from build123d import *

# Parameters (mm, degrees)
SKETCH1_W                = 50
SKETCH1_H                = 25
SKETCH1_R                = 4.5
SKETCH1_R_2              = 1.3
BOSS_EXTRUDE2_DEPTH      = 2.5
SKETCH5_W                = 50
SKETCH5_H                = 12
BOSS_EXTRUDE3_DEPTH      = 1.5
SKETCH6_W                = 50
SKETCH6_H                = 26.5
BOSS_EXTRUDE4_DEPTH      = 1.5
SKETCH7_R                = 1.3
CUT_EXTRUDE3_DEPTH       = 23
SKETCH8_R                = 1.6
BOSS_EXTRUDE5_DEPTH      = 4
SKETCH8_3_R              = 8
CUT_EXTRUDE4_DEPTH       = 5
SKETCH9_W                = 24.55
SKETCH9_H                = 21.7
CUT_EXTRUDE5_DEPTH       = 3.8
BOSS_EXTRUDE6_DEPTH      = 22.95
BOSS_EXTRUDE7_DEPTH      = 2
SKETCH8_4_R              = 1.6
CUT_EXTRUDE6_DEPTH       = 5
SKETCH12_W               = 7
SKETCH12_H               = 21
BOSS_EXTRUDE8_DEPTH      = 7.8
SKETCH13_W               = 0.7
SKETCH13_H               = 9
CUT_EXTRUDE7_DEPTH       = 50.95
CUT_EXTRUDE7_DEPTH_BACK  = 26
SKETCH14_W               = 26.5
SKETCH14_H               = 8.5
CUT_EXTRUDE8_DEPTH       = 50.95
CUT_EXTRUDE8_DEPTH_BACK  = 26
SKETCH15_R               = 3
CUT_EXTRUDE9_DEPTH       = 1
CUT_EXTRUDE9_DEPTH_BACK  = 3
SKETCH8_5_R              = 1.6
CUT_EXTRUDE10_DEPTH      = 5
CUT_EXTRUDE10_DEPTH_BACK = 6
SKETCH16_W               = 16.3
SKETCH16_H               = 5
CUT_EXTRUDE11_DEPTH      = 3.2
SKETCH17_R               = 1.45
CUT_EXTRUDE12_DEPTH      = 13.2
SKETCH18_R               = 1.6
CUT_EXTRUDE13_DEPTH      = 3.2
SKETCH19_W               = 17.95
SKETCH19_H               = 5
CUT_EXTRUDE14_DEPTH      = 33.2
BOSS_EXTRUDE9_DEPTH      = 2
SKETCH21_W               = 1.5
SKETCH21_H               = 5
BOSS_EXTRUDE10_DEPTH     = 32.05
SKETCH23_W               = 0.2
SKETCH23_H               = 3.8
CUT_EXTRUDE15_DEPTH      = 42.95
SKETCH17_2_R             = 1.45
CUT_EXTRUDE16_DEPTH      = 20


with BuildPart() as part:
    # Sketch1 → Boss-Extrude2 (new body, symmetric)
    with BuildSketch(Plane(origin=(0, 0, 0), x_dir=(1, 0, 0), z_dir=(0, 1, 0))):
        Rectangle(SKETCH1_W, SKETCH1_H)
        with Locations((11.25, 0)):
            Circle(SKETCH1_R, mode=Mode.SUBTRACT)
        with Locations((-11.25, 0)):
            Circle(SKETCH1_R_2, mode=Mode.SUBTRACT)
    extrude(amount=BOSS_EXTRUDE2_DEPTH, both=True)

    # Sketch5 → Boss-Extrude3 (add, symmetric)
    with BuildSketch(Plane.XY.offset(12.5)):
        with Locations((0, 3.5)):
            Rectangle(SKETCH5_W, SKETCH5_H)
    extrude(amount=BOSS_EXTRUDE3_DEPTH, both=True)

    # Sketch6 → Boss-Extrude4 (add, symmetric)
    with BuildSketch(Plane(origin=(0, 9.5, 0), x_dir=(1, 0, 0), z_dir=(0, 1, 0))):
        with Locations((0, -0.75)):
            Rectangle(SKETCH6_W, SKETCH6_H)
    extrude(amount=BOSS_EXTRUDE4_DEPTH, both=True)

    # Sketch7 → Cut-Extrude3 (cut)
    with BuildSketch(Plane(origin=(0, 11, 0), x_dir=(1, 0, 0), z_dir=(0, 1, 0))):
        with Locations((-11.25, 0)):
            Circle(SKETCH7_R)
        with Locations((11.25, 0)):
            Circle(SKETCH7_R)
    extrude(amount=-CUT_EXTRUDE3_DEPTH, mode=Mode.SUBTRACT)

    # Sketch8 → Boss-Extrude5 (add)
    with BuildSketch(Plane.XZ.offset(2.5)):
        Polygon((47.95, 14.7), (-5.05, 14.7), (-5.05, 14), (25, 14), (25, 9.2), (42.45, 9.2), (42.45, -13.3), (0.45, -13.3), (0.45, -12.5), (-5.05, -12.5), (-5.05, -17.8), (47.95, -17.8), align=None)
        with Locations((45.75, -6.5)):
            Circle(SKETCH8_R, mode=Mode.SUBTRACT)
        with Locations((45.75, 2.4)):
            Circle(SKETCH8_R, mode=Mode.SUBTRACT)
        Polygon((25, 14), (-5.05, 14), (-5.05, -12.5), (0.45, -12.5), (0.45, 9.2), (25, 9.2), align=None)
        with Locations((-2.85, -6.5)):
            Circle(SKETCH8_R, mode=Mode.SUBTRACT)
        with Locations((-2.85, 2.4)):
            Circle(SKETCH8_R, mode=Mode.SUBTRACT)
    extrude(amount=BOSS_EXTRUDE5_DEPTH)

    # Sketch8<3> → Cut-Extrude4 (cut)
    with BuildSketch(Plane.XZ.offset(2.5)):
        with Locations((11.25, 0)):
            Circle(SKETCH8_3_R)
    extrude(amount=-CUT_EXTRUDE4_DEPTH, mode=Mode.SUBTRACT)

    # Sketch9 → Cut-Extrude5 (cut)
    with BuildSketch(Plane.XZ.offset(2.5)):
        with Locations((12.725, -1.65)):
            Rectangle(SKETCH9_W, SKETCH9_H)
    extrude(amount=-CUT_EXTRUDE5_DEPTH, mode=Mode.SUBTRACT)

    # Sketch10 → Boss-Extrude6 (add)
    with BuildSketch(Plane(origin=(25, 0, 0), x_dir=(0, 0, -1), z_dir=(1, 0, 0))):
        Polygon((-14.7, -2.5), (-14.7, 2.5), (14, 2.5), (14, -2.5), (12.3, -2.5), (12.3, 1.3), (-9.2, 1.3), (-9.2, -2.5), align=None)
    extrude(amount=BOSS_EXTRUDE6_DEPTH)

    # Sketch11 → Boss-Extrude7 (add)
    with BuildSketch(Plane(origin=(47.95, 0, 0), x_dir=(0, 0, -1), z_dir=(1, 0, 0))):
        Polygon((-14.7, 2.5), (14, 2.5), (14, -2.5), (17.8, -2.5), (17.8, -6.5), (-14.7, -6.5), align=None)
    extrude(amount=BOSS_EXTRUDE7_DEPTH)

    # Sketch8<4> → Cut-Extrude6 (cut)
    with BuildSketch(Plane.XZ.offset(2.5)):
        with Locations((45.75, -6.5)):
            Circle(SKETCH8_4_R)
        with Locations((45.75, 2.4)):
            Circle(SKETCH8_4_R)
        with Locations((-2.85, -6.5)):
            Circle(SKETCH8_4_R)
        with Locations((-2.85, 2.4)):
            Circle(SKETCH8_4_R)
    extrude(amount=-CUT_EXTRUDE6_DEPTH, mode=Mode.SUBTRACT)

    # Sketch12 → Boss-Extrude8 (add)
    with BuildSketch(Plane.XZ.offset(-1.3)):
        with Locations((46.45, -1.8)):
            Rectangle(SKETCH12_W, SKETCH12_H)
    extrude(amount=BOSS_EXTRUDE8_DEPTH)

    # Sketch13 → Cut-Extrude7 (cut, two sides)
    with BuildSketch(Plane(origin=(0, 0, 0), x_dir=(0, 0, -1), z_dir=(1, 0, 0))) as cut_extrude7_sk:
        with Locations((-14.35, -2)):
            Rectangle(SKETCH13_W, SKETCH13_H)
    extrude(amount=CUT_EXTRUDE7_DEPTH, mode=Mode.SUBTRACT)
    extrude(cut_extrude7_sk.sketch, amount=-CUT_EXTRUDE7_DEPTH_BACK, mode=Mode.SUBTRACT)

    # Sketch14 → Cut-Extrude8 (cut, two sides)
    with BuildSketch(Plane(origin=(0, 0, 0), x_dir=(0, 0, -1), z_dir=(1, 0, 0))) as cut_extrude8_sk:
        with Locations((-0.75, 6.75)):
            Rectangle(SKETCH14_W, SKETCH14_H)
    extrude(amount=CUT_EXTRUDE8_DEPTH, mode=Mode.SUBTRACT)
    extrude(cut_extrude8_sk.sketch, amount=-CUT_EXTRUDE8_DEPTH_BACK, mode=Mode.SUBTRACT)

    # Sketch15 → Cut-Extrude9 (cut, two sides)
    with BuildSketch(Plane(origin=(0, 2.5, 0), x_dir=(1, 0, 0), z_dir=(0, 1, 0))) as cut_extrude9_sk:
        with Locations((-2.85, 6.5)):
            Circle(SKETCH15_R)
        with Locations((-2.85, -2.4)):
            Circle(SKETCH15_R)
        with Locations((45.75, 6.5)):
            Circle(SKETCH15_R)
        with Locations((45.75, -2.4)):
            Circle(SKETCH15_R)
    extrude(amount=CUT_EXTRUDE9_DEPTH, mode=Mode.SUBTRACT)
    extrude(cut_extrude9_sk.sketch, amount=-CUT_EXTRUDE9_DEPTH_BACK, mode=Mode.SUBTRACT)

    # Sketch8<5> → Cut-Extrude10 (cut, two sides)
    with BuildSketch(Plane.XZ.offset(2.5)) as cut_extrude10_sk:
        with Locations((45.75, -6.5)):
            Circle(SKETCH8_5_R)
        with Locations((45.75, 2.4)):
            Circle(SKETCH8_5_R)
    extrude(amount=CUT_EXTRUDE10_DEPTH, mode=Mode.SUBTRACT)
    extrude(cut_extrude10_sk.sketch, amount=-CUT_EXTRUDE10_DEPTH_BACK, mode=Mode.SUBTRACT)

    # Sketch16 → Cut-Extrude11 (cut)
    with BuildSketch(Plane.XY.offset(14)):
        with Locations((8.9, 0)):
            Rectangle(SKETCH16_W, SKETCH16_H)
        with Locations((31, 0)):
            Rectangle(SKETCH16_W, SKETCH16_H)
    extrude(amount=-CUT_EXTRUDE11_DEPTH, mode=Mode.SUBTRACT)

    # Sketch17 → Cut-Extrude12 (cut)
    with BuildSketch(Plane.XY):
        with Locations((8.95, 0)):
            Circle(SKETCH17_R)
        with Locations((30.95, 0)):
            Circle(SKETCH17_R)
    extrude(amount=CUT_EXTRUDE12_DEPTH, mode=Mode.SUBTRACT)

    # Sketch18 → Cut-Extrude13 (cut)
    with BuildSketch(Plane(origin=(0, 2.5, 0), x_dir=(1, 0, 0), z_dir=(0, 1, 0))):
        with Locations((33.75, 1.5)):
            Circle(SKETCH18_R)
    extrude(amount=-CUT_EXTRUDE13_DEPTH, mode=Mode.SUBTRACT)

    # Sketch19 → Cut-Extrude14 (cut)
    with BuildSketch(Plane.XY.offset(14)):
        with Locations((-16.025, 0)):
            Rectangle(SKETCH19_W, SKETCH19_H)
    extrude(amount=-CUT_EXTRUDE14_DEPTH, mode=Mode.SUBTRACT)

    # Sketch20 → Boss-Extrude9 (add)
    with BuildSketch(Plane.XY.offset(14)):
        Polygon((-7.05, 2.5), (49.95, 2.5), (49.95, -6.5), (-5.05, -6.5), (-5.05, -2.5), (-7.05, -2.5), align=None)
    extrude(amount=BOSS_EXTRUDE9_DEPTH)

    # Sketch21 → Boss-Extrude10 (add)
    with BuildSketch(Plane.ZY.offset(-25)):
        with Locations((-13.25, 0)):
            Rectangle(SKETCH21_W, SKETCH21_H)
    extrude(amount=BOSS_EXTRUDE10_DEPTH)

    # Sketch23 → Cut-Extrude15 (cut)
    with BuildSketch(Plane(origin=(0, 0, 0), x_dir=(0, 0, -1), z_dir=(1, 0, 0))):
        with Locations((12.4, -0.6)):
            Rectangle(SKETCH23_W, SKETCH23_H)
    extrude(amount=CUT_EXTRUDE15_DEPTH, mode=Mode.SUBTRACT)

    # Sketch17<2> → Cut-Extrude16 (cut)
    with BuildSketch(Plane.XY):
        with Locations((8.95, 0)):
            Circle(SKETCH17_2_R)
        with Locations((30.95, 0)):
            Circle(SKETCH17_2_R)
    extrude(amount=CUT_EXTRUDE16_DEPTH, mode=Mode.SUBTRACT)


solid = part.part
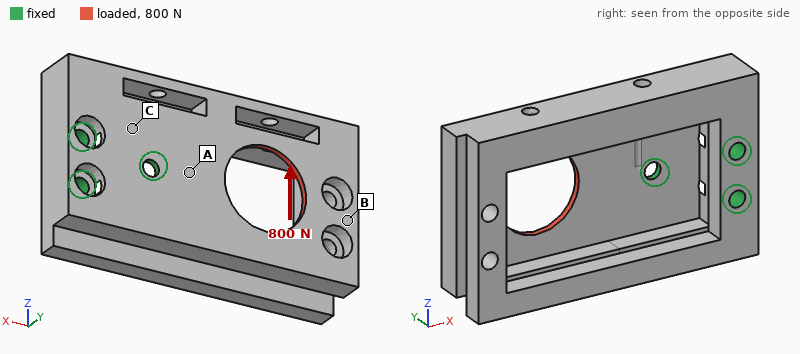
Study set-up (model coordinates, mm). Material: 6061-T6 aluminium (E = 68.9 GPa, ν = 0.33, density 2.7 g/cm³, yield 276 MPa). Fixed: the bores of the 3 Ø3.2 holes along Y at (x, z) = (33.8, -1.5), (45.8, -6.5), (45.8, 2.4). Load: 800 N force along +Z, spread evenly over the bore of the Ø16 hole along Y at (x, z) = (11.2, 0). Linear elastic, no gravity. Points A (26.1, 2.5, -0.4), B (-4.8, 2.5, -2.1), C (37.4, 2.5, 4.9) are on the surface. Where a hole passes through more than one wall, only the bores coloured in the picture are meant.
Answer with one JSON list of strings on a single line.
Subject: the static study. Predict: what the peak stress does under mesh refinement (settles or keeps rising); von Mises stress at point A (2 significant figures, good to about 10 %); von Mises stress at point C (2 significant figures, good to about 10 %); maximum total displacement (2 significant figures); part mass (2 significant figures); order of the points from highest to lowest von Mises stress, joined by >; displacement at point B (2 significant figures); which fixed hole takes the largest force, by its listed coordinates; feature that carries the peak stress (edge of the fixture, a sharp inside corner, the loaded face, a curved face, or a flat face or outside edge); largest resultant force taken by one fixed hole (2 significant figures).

["keeps rising", "62 MPa", "37 MPa", "0.13 mm", "20 g", "A > C > B", "0.098 mm", "(33.8, -1.5)", "edge of the fixture", "1.2 kN"]
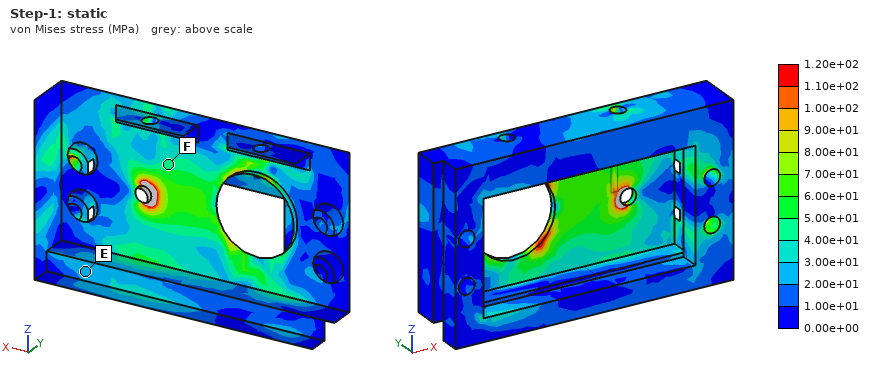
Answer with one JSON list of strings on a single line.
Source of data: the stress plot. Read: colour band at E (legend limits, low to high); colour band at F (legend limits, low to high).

["2.00e+01 to 3.00e+01 MPa", "4.00e+01 to 5.00e+01 MPa"]
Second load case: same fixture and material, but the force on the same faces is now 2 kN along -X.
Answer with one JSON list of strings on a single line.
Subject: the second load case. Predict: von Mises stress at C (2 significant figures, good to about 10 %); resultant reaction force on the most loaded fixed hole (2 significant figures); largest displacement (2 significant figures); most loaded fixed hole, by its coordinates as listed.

["52 MPa", "1.3 kN", "0.15 mm", "(33.8, -1.5)"]
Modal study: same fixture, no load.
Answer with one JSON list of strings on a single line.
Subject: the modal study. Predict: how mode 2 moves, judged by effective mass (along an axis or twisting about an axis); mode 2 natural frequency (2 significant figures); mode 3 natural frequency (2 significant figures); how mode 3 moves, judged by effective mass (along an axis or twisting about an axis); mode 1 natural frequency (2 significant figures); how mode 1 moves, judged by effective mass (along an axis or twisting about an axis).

["along Z", "2800 Hz", "4800 Hz", "along Z", "1900 Hz", "along Y"]
